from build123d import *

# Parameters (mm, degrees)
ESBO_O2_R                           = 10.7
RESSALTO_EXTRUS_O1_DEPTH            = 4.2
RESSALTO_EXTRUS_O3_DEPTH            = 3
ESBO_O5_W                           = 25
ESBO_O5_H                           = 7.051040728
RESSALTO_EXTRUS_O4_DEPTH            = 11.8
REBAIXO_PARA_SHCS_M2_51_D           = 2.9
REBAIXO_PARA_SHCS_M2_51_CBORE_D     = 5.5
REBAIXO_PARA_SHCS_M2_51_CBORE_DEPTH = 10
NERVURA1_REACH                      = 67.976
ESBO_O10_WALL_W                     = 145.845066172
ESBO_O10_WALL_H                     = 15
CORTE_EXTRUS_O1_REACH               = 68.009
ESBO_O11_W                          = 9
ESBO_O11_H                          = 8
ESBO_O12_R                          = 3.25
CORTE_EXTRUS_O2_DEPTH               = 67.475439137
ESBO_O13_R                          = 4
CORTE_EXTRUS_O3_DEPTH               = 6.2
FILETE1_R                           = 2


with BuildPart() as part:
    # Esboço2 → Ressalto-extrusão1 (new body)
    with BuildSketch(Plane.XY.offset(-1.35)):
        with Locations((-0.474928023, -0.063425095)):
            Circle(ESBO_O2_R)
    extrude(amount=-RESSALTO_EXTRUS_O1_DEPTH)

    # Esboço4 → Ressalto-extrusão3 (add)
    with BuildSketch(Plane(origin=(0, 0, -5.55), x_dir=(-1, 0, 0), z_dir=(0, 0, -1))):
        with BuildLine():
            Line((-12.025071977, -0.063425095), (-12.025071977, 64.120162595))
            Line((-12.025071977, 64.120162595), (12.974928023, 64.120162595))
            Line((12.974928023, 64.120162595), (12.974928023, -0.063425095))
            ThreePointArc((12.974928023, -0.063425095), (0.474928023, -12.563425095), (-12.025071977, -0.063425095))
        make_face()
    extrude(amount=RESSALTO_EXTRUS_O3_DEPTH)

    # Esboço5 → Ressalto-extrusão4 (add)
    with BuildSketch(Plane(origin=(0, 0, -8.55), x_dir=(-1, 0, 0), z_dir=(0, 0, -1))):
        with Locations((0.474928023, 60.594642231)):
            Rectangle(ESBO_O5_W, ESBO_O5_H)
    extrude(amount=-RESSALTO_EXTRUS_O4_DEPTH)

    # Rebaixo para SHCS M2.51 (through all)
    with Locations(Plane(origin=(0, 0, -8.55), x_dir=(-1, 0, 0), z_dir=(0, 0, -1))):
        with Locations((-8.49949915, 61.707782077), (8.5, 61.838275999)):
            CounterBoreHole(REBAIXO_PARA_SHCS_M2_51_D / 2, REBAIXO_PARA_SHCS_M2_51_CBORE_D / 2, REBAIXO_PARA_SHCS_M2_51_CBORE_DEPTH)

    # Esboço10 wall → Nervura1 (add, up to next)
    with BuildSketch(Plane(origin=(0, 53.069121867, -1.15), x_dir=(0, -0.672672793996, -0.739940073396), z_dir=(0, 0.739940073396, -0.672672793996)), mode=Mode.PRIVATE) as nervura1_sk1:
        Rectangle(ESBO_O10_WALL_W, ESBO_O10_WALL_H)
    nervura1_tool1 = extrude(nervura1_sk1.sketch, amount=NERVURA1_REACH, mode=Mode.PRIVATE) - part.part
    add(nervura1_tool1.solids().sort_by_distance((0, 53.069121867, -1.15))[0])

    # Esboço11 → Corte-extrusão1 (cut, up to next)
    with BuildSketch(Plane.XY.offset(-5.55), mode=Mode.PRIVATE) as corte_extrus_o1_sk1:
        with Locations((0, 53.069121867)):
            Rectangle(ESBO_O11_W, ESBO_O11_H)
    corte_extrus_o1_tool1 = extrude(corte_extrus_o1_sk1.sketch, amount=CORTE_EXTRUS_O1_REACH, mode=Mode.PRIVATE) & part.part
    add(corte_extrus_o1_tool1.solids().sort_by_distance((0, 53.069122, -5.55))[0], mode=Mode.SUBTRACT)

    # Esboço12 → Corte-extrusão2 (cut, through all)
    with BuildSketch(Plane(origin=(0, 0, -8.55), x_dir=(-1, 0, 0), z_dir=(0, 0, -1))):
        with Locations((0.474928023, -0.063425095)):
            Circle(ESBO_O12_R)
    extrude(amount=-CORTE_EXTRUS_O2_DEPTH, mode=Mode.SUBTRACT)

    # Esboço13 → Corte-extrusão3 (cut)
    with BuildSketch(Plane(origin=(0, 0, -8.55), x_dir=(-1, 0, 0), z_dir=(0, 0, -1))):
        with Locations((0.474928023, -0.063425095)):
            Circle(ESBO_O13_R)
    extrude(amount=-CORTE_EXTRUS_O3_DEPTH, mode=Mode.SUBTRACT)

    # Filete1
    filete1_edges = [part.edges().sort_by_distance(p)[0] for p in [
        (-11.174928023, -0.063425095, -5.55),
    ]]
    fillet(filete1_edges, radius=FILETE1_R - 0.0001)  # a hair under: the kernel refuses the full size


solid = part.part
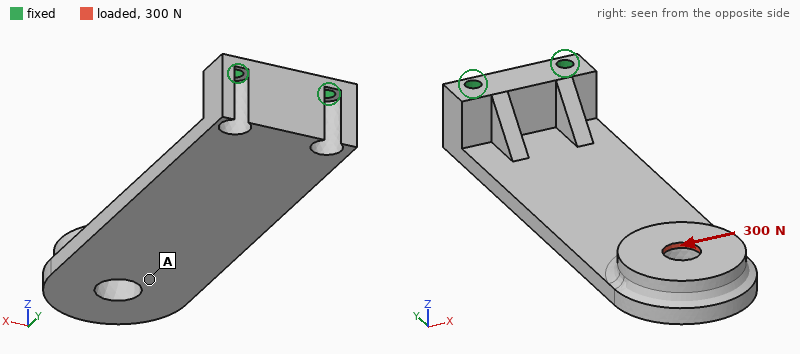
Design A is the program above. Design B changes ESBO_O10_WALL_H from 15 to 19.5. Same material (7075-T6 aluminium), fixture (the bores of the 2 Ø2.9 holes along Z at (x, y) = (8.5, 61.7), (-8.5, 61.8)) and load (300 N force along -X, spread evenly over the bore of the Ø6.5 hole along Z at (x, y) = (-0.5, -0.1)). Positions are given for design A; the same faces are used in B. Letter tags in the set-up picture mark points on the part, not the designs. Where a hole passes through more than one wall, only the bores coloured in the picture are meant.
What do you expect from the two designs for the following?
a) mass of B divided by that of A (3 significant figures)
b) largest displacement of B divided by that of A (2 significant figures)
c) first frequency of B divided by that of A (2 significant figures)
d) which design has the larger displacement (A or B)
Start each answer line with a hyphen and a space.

- 1.02
- 0.86
- 1.0
- A
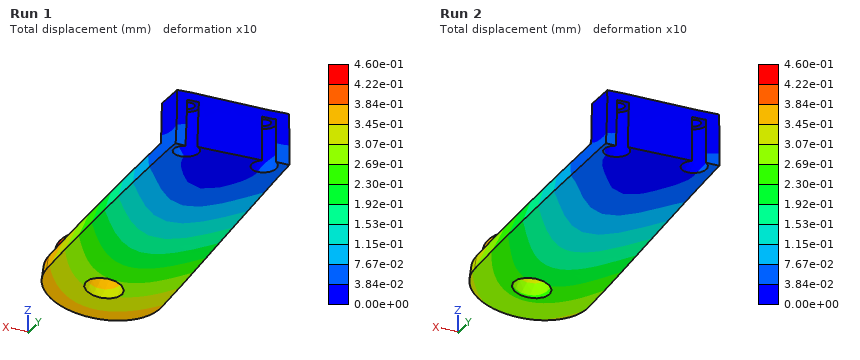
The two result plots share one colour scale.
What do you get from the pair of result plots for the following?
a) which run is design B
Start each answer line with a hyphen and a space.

- Run 2
